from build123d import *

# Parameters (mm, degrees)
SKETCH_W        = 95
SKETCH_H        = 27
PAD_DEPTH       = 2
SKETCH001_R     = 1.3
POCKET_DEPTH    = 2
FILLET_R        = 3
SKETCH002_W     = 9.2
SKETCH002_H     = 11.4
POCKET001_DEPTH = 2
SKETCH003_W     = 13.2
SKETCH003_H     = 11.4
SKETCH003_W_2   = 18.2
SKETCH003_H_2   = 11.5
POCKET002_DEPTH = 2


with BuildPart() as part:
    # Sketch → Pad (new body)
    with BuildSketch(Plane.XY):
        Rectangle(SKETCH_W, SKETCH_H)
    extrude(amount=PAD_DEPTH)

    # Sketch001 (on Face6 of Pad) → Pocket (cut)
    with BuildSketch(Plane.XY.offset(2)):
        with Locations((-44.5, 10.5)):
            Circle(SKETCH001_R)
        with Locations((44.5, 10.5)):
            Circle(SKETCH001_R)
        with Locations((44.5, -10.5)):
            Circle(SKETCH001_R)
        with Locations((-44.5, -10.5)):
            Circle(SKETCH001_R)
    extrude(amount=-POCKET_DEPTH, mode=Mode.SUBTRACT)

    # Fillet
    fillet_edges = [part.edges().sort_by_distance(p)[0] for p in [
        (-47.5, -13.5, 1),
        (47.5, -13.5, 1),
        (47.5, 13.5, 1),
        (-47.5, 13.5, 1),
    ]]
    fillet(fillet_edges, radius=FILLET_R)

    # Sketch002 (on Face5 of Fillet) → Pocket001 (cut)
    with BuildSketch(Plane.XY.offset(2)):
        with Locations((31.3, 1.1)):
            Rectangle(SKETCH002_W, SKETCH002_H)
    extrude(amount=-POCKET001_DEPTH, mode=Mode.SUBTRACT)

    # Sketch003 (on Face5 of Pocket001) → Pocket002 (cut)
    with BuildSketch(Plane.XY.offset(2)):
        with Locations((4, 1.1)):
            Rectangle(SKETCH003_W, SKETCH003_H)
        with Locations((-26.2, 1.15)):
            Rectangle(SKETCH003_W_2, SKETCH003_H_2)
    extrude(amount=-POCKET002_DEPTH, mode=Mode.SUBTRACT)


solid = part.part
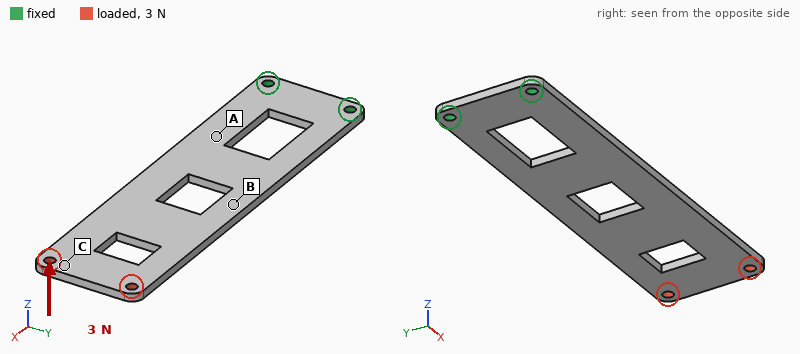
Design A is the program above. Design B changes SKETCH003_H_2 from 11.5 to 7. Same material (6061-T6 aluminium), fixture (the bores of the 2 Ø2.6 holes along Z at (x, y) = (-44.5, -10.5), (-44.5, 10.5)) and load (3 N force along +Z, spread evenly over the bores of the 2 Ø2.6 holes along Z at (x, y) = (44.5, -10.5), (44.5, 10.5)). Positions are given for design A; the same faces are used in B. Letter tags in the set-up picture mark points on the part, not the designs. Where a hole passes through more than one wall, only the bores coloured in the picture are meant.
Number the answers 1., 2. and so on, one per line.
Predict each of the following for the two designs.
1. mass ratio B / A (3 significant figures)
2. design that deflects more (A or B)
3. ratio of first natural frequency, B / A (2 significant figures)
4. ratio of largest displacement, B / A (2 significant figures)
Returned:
1. 1.04
2. A
3. 1.1
4. 0.86
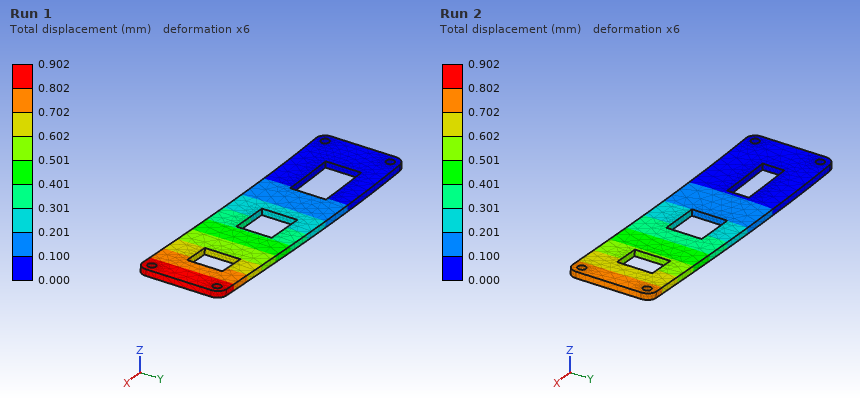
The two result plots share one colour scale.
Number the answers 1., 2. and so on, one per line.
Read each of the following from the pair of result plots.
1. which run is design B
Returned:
1. Run 2
